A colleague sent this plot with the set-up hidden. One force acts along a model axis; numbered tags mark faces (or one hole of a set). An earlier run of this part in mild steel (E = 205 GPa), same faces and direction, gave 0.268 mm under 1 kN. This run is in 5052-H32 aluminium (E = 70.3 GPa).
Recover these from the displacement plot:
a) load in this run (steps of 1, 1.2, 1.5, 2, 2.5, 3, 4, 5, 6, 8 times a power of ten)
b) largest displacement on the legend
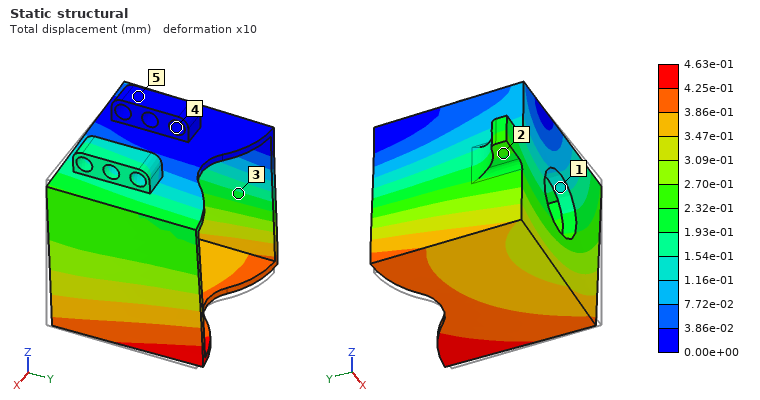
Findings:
600 N
4.63e-01 mm
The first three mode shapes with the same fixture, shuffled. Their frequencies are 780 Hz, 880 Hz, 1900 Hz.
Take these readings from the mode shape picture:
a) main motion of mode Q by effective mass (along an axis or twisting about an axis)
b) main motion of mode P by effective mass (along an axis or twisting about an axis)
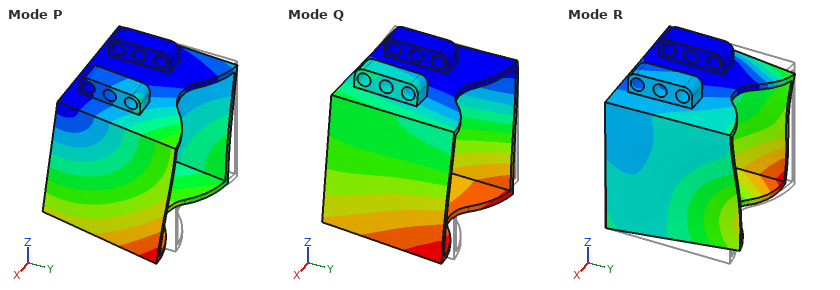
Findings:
along X
along Y
